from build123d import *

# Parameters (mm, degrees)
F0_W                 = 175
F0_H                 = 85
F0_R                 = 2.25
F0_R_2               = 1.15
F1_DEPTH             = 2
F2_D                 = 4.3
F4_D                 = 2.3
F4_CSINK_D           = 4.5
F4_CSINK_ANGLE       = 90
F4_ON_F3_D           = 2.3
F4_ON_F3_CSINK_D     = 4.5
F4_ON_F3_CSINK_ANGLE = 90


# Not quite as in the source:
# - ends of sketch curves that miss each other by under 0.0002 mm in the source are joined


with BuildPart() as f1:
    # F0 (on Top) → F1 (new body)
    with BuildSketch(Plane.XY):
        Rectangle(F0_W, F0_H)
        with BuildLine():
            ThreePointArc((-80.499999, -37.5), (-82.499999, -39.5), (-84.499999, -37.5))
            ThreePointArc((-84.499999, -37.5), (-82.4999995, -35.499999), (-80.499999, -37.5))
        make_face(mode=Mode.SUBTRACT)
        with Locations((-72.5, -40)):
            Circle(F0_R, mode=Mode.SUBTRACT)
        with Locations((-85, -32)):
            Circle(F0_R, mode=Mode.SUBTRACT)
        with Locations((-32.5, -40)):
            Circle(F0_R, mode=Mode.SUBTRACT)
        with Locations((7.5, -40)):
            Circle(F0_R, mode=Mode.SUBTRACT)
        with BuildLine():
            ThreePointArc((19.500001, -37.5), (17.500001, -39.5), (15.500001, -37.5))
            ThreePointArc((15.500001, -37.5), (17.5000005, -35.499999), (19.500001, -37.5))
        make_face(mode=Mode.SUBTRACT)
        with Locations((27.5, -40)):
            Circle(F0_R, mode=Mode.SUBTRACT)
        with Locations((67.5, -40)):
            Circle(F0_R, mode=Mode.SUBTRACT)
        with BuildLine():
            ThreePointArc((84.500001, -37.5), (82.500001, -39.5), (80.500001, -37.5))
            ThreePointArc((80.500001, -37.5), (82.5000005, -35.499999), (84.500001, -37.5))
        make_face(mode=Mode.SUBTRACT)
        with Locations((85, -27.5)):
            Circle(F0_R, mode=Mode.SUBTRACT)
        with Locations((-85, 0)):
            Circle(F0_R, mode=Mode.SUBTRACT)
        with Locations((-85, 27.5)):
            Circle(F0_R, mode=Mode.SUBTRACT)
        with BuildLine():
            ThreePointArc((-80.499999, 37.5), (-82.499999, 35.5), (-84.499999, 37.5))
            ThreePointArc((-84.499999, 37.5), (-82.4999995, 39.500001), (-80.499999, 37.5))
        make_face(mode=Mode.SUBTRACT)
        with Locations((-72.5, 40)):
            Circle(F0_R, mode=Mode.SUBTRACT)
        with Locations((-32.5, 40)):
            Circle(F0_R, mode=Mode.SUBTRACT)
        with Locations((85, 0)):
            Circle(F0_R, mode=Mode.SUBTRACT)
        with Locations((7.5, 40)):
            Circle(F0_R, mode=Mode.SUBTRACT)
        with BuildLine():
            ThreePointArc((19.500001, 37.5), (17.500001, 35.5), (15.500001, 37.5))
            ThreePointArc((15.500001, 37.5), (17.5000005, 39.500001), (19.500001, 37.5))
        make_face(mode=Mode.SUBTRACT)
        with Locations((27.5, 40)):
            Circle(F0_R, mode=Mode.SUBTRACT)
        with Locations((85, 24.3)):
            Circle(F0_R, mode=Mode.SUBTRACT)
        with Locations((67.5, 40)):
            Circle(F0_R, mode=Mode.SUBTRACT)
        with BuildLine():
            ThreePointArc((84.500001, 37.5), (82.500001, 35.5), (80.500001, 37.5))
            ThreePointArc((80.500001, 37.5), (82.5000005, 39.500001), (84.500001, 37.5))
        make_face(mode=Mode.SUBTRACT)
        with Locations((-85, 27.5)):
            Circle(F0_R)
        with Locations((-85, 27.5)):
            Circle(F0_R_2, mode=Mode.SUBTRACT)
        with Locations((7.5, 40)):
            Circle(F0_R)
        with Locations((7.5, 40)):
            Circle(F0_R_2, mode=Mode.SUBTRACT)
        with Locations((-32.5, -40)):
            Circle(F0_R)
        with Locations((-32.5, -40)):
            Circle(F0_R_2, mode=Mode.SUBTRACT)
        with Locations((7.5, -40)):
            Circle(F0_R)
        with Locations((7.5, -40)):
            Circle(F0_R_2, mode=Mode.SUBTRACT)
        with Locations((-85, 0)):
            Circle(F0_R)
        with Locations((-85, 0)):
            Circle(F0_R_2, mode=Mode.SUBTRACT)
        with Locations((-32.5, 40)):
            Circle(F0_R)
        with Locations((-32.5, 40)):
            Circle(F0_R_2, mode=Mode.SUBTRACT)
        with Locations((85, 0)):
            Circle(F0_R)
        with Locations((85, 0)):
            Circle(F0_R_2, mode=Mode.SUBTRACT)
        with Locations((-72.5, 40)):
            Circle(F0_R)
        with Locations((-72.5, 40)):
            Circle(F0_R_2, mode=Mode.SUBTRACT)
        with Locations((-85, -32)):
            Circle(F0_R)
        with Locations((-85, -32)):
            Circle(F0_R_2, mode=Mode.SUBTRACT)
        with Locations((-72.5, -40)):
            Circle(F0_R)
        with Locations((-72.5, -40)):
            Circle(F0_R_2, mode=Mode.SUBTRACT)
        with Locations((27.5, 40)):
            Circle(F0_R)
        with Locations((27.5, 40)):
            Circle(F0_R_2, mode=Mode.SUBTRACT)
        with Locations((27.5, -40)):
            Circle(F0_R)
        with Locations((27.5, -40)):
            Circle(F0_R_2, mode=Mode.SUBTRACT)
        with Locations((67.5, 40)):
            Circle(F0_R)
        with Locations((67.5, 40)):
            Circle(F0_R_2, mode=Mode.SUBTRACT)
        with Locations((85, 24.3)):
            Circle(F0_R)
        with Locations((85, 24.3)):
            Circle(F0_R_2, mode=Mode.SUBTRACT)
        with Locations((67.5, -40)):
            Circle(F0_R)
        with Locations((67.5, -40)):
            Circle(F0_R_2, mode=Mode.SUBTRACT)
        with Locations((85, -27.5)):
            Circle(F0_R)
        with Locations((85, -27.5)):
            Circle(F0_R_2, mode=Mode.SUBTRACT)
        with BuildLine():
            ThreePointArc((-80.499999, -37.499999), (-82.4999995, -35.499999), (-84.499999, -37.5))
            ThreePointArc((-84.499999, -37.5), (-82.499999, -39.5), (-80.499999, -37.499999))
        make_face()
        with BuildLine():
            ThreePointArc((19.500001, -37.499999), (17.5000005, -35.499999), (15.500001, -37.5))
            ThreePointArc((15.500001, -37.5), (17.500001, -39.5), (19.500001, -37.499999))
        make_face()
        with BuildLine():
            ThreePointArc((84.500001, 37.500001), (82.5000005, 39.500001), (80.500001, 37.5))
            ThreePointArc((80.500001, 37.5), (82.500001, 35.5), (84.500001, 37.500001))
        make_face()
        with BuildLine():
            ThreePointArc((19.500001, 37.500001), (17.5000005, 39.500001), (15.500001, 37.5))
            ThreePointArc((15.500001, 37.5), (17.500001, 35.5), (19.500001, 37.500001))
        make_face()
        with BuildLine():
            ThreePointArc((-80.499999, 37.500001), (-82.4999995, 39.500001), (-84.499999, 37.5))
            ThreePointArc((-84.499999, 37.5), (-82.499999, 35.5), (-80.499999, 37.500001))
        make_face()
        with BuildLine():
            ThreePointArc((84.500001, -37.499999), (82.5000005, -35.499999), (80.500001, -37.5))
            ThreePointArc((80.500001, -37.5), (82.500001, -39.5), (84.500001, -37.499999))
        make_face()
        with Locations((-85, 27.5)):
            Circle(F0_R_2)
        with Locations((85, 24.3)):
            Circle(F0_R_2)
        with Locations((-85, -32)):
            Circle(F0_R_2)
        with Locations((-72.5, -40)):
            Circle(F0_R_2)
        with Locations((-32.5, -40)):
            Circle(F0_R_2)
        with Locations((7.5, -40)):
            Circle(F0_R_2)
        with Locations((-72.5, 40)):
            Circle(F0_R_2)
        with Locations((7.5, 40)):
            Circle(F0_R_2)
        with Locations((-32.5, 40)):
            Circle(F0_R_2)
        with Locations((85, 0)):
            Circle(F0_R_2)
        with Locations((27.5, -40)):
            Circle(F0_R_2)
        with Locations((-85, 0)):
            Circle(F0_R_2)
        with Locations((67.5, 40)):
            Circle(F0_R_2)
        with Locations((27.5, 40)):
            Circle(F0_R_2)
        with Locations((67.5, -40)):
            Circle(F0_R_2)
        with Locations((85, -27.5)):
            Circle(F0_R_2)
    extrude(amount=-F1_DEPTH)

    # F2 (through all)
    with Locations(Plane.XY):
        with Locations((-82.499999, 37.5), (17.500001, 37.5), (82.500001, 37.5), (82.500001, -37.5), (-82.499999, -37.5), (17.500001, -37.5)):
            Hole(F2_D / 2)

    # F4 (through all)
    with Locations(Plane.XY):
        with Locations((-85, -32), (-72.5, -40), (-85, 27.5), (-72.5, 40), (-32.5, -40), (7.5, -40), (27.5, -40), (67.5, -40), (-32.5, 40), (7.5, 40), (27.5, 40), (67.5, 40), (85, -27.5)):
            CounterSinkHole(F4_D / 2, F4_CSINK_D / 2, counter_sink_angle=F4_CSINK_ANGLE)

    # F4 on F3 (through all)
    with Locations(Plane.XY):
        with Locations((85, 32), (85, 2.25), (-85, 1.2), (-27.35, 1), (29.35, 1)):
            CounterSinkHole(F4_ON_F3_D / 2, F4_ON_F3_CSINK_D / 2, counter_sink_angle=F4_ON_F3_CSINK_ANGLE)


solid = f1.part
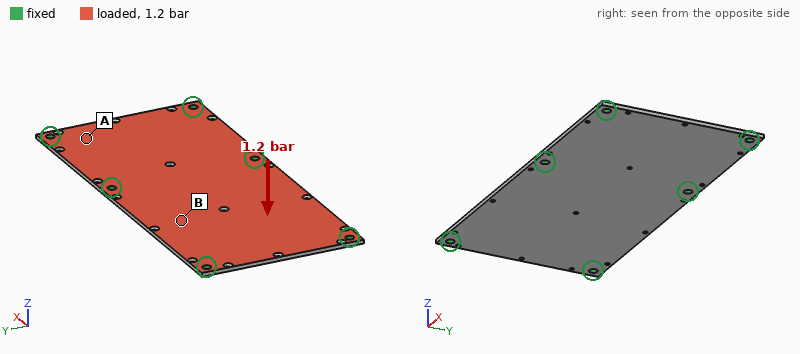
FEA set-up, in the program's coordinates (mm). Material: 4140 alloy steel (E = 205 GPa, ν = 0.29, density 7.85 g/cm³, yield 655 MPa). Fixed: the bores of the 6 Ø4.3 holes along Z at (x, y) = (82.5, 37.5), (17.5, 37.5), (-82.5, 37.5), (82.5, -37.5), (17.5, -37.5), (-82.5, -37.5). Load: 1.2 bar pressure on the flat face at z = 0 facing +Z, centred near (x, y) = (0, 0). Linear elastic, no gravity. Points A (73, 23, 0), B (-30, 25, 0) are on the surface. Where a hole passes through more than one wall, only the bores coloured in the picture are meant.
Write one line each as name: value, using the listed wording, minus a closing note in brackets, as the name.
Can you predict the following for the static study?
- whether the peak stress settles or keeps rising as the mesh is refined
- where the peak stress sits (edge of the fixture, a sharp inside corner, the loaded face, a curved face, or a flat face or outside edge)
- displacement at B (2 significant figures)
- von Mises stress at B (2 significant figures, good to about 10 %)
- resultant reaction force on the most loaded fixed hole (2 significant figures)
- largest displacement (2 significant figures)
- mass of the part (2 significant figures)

whether the peak stress settles or keeps rising as the mesh is refined: keeps rising
where the peak stress sits: edge of the fixture
displacement at B: 0.34 mm
von Mises stress at B: 84 MPa
resultant reaction force on the most loaded fixed hole: 440 N
largest displacement: 0.39 mm
mass of the part: 230 g
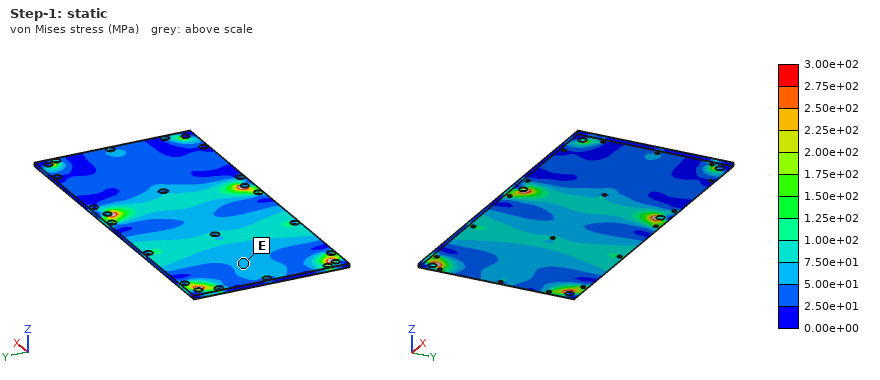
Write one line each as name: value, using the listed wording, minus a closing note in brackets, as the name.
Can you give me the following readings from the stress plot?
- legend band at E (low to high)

legend band at E: 5.00e+01 to 7.50e+01 MPa
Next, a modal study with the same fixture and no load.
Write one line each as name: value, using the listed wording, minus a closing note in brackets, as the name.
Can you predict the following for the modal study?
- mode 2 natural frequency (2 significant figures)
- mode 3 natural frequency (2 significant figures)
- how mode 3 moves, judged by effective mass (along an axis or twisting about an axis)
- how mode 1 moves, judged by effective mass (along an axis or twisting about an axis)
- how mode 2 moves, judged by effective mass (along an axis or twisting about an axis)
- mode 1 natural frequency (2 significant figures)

mode 2 natural frequency: 1300 Hz
mode 3 natural frequency: 1400 Hz
how mode 3 moves, judged by effective mass: along Z
how mode 1 moves, judged by effective mass: along Z
how mode 2 moves, judged by effective mass: twisting about X
mode 1 natural frequency: 820 Hz
